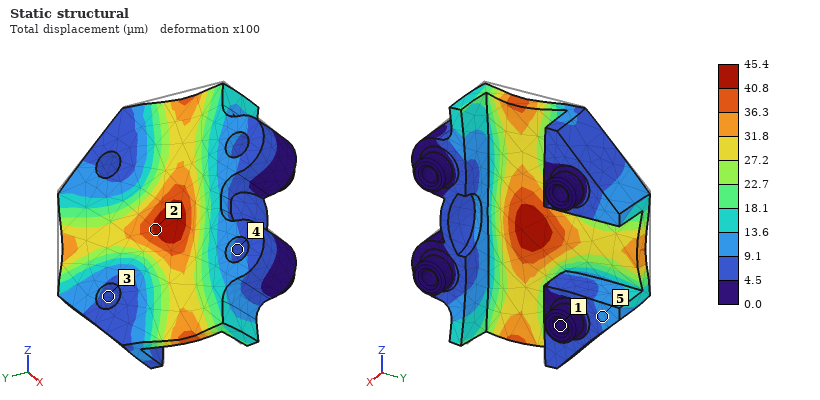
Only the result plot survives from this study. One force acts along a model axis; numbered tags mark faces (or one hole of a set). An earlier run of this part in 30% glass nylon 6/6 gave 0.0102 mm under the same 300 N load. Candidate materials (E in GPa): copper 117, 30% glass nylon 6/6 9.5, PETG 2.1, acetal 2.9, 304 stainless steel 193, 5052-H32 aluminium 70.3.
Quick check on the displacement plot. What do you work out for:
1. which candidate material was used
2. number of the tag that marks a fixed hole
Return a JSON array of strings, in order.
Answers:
["PETG", "1"]
